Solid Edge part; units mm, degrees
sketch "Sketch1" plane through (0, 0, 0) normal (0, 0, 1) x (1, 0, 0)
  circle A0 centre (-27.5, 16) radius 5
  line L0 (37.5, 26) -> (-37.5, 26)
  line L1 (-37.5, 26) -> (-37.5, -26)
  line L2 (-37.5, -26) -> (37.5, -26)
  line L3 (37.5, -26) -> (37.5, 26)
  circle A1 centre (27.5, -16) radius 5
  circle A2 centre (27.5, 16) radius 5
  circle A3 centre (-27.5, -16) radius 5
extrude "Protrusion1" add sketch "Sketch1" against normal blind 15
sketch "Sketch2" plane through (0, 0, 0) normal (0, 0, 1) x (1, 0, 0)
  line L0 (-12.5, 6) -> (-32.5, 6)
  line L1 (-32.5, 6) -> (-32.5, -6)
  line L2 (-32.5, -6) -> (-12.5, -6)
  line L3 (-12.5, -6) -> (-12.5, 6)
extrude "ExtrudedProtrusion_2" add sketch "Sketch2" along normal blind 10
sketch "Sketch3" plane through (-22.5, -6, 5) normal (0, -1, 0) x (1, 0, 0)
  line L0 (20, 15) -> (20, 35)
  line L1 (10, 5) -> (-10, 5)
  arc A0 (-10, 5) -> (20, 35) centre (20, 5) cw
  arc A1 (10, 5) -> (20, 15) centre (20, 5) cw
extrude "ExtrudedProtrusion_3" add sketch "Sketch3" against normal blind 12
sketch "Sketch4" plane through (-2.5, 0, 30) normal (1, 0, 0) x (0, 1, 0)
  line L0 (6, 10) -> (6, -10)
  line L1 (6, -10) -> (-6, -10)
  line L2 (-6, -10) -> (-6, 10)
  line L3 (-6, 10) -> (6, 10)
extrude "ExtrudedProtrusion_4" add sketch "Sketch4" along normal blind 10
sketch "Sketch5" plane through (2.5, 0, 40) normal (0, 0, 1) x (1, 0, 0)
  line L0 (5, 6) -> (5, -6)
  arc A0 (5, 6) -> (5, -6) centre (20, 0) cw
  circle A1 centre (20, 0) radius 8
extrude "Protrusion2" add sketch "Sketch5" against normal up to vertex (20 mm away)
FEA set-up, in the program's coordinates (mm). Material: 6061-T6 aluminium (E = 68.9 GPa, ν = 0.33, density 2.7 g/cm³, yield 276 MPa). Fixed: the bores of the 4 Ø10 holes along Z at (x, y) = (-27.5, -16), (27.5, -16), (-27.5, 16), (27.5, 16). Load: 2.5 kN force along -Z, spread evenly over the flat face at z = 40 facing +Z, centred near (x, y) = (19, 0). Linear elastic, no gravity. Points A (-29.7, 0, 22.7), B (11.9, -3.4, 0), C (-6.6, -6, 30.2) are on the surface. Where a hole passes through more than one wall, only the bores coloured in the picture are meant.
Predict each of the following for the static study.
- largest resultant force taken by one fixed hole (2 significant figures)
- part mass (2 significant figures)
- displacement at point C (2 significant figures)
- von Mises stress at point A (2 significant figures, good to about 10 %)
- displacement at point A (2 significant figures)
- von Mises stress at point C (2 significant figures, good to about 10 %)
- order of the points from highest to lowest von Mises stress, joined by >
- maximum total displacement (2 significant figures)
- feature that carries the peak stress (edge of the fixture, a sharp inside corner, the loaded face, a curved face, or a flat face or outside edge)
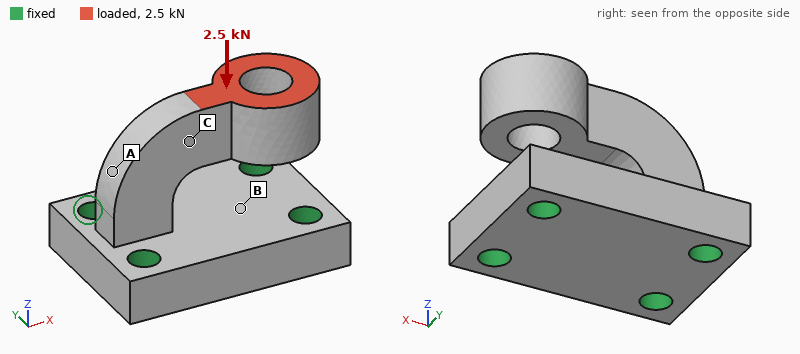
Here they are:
710 N
210 g
0.17 mm
83 MPa
0.087 mm
33 MPa
A > C > B
0.57 mm
a curved face
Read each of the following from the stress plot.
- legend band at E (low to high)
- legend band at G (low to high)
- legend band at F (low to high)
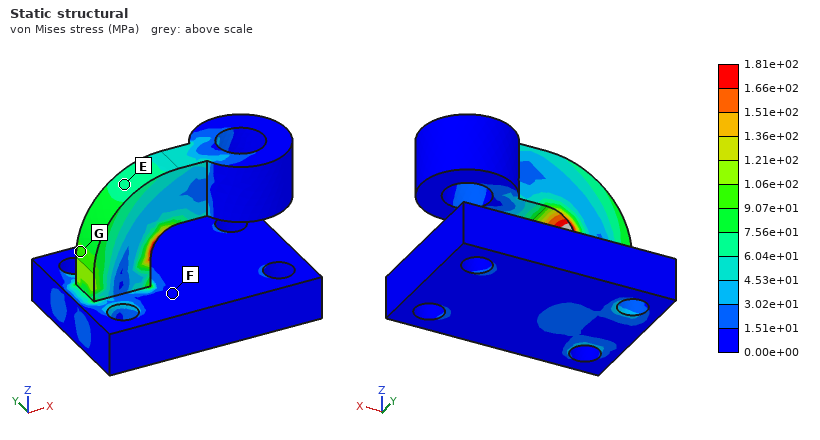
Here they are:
6.04e+01 to 7.56e+01 MPa
9.07e+01 to 1.06e+02 MPa
0.00e+00 to 1.51e+01 MPa
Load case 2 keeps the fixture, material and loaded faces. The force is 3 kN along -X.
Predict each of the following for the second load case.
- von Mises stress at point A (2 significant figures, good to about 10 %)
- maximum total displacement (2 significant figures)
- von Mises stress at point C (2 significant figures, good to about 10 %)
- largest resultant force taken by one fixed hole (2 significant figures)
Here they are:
63 MPa
0.48 mm
26 MPa
1.5 kN
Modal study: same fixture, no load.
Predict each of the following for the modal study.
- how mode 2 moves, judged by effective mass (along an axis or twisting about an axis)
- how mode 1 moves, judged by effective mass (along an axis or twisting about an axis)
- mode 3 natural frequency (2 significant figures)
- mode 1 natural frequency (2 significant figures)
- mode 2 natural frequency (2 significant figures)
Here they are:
along Z
along Y
3800 Hz
1200 Hz
1900 Hz
